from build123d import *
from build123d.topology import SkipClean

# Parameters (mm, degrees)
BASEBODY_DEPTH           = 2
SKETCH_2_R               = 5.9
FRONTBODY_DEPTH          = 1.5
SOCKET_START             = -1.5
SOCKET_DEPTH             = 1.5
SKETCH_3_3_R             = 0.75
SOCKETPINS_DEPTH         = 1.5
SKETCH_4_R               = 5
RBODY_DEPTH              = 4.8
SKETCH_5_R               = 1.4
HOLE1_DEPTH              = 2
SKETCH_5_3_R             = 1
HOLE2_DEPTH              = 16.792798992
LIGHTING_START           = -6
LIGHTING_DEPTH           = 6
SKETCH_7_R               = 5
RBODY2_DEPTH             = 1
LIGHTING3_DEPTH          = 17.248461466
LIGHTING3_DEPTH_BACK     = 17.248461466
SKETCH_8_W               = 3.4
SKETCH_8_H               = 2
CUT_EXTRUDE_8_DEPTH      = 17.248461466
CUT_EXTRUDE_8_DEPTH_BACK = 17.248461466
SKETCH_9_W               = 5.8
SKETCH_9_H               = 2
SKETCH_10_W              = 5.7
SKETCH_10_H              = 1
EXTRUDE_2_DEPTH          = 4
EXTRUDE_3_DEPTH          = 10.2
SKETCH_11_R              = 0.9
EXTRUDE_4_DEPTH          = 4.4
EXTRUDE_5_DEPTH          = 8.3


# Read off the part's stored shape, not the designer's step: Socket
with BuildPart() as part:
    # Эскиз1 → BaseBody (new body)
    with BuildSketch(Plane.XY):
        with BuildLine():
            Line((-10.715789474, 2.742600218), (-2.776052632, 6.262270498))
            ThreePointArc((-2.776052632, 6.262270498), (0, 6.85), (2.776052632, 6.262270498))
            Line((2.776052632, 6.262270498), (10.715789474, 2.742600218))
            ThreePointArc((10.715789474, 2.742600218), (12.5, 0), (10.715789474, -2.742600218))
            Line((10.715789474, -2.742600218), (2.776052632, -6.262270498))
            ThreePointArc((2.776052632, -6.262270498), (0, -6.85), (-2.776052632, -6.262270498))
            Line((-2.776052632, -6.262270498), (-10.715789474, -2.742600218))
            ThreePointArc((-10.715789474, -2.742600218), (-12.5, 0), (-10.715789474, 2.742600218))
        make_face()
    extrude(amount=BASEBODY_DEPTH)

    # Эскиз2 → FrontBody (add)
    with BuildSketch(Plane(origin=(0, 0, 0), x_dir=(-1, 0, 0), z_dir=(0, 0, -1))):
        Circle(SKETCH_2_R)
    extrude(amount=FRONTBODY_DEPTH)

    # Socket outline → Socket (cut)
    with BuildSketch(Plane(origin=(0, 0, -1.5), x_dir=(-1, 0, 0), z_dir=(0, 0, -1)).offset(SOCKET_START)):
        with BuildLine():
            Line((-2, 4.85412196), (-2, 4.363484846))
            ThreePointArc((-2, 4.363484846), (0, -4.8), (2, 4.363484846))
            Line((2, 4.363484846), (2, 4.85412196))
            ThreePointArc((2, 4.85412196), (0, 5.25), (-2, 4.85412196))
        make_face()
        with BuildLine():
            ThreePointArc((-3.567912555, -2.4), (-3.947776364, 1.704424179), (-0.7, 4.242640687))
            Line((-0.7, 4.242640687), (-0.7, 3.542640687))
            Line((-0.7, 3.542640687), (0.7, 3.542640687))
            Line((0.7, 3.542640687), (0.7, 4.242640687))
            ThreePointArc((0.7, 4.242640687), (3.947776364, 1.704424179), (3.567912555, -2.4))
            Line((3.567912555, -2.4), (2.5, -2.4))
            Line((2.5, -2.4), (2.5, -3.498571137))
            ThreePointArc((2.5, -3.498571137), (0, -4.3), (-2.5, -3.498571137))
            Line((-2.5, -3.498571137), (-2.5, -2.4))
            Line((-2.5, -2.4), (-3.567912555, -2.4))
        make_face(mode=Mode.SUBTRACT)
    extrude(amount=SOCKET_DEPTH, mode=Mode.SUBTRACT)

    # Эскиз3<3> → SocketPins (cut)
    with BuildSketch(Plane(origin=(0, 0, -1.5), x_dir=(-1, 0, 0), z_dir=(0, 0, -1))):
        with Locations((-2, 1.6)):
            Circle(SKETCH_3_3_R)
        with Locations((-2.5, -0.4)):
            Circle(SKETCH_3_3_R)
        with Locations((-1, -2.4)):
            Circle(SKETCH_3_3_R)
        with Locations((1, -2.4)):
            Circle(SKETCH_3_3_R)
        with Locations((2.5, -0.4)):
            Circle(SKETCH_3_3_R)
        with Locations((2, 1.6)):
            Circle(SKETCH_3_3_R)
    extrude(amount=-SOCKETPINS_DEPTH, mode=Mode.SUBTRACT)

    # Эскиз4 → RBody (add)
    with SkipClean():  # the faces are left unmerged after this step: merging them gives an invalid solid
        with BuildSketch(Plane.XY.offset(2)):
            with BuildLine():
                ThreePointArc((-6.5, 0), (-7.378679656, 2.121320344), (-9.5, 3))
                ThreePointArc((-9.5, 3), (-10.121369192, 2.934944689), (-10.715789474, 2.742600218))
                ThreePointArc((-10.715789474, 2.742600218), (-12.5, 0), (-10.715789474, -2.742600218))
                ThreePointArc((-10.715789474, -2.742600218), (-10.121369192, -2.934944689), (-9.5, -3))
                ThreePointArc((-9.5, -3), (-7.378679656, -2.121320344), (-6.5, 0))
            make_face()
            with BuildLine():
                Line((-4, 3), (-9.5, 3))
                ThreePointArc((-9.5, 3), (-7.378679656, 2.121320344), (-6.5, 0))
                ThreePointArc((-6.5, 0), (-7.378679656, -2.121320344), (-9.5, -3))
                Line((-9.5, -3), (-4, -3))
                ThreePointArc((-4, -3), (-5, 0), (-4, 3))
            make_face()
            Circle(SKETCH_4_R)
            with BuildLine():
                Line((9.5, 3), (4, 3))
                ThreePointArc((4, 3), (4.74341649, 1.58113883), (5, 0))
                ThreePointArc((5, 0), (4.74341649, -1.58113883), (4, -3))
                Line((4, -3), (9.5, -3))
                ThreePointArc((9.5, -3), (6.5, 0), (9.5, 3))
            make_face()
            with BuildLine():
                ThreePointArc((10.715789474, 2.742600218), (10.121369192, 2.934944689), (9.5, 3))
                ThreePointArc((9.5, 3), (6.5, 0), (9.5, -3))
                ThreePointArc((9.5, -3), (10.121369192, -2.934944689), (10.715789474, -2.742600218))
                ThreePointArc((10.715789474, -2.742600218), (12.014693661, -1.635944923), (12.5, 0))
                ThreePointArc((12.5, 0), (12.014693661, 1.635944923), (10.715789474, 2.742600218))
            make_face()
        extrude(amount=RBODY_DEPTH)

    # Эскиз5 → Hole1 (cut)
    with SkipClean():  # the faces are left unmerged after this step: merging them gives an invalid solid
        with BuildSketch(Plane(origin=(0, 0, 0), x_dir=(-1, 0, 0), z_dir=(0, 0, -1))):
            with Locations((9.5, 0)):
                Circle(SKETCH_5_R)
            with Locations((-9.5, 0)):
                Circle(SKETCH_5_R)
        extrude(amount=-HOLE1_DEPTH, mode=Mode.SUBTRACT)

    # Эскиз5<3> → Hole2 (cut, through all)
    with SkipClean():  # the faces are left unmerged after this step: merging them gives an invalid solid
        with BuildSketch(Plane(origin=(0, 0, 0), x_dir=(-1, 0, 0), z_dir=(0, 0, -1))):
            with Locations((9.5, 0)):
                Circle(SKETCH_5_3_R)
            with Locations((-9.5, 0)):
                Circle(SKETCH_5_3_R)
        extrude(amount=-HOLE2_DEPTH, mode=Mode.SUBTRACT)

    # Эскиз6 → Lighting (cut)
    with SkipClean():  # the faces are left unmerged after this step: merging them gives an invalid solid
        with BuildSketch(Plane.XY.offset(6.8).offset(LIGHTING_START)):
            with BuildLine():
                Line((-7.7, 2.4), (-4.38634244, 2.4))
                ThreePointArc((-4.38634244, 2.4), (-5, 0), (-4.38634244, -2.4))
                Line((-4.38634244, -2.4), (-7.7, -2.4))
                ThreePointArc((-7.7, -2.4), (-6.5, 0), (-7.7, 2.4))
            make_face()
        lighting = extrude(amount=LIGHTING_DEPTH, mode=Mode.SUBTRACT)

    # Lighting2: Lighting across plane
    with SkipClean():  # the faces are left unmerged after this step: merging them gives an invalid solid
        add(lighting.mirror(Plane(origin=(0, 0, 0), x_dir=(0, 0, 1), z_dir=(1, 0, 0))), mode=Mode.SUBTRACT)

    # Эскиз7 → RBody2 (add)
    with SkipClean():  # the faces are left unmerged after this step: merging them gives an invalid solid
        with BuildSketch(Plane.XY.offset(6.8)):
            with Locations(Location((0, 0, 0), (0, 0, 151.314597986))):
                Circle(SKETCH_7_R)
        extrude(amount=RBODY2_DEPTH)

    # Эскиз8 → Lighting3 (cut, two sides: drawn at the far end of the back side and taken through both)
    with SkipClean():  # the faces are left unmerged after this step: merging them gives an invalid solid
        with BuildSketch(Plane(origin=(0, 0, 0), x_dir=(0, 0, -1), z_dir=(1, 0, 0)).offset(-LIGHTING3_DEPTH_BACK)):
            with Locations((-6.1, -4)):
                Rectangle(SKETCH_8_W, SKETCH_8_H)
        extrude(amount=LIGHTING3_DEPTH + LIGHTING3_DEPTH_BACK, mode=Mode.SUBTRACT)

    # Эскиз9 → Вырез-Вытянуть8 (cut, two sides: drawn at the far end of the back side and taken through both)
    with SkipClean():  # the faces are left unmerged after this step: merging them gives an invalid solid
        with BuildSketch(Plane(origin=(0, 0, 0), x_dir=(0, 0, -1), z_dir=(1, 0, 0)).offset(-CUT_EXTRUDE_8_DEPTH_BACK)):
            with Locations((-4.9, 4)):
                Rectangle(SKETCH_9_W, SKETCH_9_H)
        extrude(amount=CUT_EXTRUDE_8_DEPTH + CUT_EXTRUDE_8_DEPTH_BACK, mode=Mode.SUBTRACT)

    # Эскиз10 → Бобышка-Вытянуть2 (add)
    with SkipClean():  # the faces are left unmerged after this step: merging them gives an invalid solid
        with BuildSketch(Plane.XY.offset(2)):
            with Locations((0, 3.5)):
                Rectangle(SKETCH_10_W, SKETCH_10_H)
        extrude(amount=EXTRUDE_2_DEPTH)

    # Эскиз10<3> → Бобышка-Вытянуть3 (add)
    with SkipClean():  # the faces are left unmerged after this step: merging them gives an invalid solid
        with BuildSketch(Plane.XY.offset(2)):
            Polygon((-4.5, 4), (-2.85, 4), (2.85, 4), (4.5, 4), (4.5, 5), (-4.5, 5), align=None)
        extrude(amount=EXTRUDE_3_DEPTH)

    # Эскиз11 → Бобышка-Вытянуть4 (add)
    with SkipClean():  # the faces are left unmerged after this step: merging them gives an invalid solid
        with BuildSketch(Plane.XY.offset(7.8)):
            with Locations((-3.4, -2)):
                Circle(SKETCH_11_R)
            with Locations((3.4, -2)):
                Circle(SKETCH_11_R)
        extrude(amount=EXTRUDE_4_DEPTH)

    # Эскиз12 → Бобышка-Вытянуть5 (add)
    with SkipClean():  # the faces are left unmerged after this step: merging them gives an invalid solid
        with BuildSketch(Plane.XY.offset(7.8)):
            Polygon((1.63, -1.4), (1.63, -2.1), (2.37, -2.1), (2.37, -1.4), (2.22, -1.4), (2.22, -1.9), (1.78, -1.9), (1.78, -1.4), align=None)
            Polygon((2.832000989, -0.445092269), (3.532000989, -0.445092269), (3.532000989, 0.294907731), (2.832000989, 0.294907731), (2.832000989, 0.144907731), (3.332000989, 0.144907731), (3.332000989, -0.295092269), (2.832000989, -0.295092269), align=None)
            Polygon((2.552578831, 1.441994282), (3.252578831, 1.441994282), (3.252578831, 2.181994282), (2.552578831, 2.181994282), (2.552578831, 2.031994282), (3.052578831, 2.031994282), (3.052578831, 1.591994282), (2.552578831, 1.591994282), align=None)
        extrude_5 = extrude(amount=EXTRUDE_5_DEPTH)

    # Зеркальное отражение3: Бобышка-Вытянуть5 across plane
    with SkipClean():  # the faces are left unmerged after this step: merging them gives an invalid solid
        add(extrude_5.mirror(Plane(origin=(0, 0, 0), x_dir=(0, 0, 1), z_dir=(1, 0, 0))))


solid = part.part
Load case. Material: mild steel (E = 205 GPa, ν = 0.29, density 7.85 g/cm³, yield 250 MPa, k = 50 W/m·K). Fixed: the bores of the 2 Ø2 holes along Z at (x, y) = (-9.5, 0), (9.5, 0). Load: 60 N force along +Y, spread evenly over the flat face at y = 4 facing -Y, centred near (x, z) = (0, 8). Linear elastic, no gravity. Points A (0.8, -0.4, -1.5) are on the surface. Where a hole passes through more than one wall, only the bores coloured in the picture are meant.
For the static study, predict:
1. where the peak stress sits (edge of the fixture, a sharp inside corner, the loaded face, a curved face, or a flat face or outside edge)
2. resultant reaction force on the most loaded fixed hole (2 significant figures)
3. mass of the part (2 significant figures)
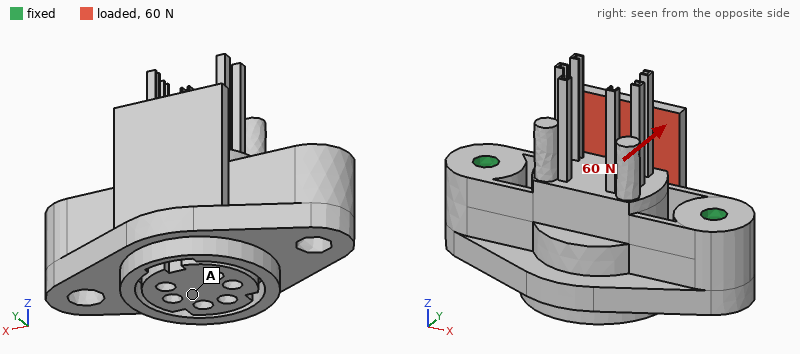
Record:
a flat face or outside edge
30 N
10 g
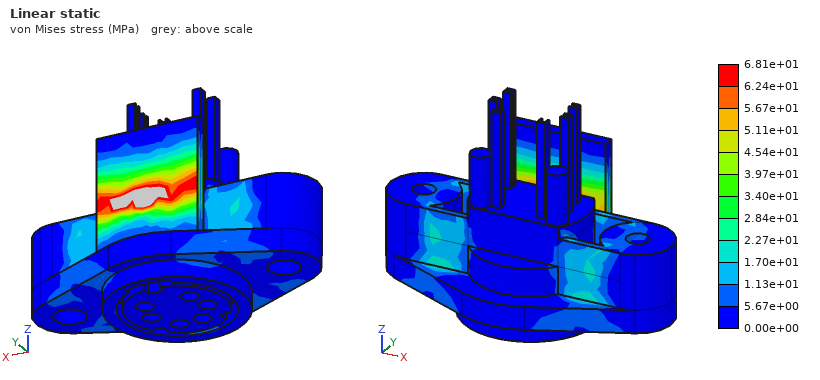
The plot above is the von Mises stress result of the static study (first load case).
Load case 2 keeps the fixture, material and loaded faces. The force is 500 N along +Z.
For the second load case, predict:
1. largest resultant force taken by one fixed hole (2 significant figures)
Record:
260 N
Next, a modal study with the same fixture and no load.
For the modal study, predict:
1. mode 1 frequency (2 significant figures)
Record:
8300 Hz
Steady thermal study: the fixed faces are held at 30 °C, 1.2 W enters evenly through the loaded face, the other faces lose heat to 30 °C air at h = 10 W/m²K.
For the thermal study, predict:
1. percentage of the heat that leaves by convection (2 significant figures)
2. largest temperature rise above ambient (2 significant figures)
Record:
4.3 %
15 K
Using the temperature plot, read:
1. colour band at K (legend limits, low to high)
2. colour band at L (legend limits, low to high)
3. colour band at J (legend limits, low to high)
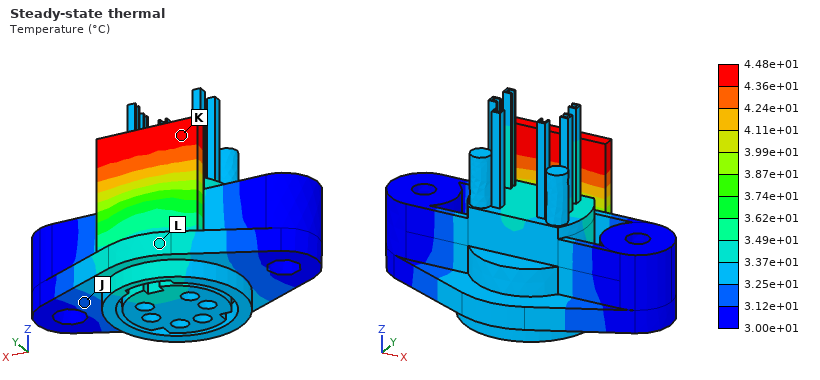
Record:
4.36e+01 to 4.48e+01 °C
3.37e+01 to 3.49e+01 °C
3.12e+01 to 3.25e+01 °C
